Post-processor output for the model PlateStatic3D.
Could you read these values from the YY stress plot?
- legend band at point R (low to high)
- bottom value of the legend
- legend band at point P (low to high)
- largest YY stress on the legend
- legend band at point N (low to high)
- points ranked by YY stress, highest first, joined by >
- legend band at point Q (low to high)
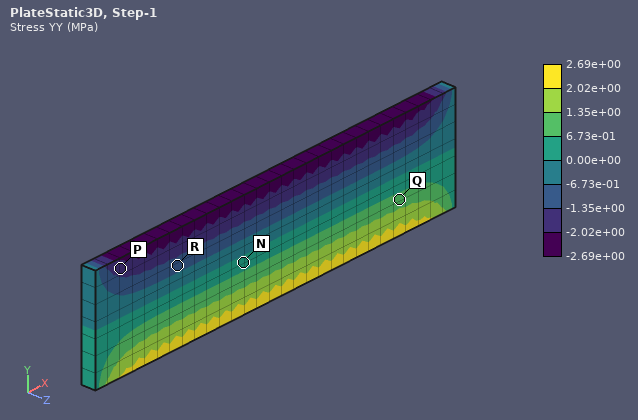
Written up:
-1.35e+00 to -6.73e-01 MPa
-2.69e+00 MPa
-2.02e+00 to -1.35e+00 MPa
2.69e+00 MPa
0.00e+00 to 6.73e-01 MPa
Q > N > R > P
6.73e-01 to 1.35e+00 MPa
